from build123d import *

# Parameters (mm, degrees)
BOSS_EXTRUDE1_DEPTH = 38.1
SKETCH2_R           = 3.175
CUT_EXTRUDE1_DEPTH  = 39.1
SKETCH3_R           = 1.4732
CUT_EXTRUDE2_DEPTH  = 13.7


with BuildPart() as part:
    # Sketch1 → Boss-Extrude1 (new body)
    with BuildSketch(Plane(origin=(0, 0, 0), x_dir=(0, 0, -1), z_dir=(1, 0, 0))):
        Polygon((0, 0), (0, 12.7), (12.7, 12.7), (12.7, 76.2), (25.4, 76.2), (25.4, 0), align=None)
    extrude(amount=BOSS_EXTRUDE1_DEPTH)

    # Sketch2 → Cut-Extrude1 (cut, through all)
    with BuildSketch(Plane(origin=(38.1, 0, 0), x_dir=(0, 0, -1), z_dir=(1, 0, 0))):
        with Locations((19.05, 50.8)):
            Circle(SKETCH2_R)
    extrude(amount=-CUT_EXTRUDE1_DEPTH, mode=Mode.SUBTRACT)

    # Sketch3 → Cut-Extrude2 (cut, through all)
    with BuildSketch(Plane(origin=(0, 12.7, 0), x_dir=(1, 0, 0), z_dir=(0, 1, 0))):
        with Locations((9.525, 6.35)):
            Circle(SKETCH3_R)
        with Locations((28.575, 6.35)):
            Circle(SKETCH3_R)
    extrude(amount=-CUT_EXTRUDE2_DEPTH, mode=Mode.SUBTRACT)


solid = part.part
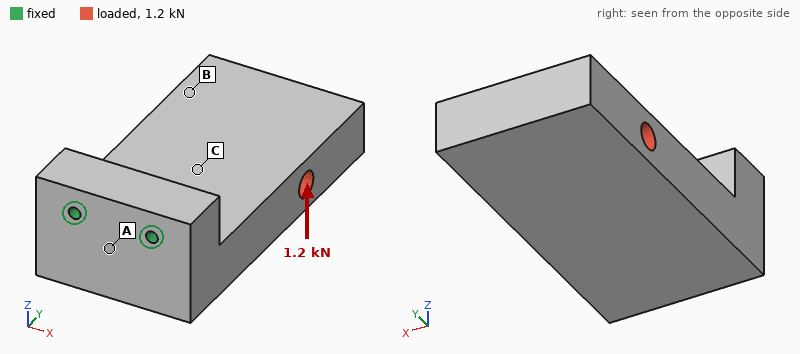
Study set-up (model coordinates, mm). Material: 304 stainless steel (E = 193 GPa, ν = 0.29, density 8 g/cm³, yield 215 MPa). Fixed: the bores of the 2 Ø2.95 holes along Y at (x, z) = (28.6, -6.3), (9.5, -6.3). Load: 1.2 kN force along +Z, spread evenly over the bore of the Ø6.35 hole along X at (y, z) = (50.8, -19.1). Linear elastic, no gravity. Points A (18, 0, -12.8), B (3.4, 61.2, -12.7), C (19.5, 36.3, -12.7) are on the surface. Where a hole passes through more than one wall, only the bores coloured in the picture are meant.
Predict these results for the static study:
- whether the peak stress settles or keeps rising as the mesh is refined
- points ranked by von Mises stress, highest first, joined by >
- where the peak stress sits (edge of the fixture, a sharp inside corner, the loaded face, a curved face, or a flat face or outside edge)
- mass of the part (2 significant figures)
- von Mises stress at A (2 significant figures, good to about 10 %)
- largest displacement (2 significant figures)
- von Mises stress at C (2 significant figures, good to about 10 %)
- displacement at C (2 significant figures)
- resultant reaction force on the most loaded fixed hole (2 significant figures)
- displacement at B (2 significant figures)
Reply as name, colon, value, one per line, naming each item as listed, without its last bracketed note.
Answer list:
whether the peak stress settles or keeps rising as the mesh is refined: keeps rising
points ranked by von Mises stress, highest first, joined by >: A > C > B
where the peak stress sits: edge of the fixture
mass of the part: 330 g
von Mises stress at A: 32 MPa
largest displacement: 90 µm
von Mises stress at C: 17 MPa
displacement at C: 31 µm
resultant reaction force on the most loaded fixed hole: 640 N
displacement at B: 67 µm
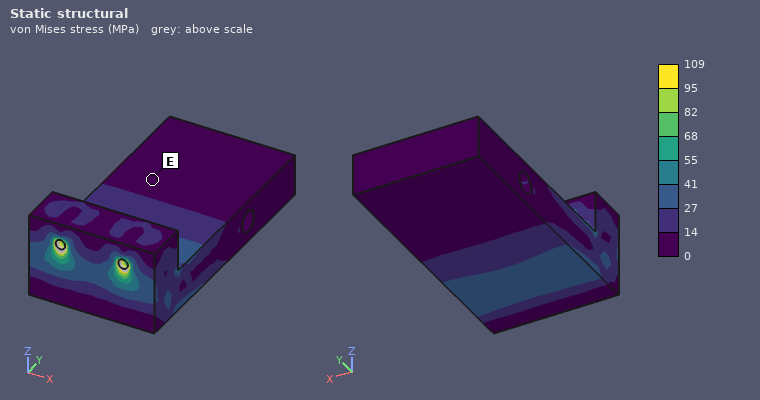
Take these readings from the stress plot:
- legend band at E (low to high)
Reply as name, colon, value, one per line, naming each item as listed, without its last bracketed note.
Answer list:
legend band at E: 0 to 14 MPa
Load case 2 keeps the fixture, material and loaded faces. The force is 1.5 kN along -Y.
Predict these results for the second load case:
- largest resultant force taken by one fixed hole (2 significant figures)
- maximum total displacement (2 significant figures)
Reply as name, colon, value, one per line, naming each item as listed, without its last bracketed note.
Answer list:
largest resultant force taken by one fixed hole: 750 N
maximum total displacement: 12 µm
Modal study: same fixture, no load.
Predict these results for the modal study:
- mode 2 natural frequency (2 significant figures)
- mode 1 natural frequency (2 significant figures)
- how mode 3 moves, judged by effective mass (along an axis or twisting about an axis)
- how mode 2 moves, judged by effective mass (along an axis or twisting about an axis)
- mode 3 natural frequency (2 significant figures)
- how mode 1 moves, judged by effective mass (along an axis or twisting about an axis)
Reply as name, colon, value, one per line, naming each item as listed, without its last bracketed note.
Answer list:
mode 2 natural frequency: 3100 Hz
mode 1 natural frequency: 1600 Hz
how mode 3 moves, judged by effective mass: twisting about Y
how mode 2 moves, judged by effective mass: along X
mode 3 natural frequency: 6600 Hz
how mode 1 moves, judged by effective mass: along Z
